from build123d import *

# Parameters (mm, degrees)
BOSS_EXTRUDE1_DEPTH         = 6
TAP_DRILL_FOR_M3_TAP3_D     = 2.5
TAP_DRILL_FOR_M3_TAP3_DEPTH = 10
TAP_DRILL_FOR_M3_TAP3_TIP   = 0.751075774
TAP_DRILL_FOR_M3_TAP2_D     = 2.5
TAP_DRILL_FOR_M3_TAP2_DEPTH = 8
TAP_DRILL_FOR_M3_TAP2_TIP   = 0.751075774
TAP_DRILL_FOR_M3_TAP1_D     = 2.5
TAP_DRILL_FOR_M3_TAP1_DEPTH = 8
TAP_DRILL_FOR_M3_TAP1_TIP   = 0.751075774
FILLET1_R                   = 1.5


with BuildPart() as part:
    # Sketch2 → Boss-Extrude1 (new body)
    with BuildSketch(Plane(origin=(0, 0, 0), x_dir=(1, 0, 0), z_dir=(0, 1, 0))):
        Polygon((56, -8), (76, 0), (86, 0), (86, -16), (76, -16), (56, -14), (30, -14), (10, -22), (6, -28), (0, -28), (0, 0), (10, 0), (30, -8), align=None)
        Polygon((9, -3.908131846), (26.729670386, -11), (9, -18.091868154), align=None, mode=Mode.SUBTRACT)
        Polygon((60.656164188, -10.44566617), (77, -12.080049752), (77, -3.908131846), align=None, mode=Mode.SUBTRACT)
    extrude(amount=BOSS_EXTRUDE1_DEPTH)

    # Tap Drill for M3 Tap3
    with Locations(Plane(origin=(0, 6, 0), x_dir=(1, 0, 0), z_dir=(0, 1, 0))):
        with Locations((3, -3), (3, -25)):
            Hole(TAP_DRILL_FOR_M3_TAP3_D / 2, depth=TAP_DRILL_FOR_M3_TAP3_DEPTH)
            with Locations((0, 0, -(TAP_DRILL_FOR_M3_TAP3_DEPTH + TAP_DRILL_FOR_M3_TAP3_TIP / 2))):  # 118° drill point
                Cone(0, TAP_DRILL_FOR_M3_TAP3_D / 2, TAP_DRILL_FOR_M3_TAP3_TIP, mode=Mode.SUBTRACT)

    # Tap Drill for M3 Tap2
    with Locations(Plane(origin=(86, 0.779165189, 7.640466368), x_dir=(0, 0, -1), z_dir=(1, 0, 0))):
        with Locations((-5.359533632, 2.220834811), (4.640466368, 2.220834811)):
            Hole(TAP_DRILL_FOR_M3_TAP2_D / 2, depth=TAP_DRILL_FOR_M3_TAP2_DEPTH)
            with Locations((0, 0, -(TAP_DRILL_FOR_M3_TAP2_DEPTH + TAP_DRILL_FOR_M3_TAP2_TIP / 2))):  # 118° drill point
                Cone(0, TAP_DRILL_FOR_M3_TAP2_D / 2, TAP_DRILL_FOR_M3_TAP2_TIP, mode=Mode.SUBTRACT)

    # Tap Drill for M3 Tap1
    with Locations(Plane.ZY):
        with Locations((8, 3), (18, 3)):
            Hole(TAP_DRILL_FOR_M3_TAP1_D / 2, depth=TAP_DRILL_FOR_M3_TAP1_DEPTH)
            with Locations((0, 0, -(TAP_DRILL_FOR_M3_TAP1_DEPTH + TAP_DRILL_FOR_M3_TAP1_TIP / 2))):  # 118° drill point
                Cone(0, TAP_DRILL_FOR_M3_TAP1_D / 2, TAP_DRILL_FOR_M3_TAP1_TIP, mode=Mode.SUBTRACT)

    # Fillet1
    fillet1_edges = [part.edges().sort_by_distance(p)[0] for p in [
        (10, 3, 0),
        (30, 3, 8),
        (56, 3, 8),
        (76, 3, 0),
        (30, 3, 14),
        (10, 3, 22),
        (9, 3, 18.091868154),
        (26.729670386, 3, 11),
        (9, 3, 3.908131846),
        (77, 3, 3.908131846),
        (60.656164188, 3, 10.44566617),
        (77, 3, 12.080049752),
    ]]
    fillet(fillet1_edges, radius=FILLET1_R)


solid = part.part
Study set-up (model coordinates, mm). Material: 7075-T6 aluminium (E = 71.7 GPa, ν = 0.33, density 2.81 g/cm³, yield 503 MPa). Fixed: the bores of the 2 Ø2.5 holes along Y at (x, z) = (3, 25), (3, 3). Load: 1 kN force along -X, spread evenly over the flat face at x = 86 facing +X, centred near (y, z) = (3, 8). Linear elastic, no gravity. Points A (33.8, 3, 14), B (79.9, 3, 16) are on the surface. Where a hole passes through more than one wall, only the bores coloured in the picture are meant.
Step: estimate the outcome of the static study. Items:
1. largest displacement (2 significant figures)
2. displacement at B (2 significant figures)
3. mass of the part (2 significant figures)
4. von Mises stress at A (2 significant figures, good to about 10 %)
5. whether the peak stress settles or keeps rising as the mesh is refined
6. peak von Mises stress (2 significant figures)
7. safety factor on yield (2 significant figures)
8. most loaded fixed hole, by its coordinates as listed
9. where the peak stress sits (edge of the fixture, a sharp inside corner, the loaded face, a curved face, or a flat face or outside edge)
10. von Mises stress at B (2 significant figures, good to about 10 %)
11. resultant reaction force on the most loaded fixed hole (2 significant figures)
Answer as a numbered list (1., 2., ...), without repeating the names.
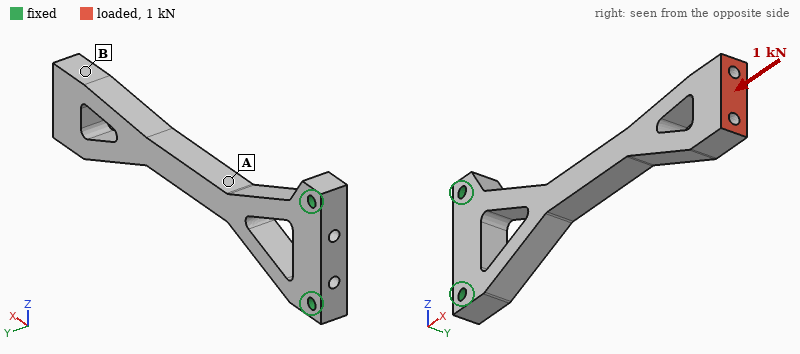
1. 0.67 mm
2. 0.55 mm
3. 15 g
4. 56 MPa
5. settles
6. 150 MPa
7. 3.4
8. (3, 3)
9. a curved face
10. 26 MPa
11. 760 N
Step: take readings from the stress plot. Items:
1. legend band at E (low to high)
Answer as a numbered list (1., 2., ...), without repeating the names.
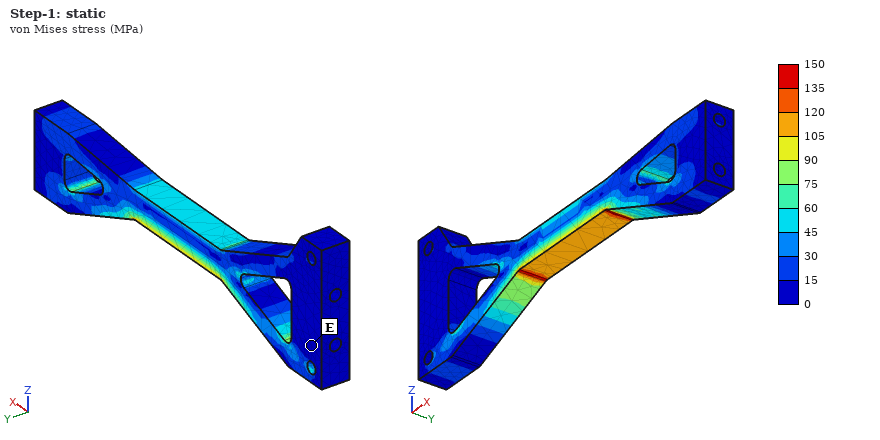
1. 0 to 15 MPa
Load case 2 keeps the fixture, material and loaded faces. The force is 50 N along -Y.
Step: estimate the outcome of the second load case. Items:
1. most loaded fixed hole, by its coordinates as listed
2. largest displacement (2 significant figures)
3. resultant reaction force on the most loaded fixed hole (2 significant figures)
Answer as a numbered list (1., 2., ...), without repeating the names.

1. (3, 3)
2. 1.0 mm
3. 38 N
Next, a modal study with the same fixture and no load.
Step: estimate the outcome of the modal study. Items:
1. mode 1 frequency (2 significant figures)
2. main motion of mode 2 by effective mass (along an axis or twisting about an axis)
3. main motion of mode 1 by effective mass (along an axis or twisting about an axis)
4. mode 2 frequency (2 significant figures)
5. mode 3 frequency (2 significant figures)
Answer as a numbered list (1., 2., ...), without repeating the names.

1. 600 Hz
2. along Z
3. along Y
4. 920 Hz
5. 4000 Hz
